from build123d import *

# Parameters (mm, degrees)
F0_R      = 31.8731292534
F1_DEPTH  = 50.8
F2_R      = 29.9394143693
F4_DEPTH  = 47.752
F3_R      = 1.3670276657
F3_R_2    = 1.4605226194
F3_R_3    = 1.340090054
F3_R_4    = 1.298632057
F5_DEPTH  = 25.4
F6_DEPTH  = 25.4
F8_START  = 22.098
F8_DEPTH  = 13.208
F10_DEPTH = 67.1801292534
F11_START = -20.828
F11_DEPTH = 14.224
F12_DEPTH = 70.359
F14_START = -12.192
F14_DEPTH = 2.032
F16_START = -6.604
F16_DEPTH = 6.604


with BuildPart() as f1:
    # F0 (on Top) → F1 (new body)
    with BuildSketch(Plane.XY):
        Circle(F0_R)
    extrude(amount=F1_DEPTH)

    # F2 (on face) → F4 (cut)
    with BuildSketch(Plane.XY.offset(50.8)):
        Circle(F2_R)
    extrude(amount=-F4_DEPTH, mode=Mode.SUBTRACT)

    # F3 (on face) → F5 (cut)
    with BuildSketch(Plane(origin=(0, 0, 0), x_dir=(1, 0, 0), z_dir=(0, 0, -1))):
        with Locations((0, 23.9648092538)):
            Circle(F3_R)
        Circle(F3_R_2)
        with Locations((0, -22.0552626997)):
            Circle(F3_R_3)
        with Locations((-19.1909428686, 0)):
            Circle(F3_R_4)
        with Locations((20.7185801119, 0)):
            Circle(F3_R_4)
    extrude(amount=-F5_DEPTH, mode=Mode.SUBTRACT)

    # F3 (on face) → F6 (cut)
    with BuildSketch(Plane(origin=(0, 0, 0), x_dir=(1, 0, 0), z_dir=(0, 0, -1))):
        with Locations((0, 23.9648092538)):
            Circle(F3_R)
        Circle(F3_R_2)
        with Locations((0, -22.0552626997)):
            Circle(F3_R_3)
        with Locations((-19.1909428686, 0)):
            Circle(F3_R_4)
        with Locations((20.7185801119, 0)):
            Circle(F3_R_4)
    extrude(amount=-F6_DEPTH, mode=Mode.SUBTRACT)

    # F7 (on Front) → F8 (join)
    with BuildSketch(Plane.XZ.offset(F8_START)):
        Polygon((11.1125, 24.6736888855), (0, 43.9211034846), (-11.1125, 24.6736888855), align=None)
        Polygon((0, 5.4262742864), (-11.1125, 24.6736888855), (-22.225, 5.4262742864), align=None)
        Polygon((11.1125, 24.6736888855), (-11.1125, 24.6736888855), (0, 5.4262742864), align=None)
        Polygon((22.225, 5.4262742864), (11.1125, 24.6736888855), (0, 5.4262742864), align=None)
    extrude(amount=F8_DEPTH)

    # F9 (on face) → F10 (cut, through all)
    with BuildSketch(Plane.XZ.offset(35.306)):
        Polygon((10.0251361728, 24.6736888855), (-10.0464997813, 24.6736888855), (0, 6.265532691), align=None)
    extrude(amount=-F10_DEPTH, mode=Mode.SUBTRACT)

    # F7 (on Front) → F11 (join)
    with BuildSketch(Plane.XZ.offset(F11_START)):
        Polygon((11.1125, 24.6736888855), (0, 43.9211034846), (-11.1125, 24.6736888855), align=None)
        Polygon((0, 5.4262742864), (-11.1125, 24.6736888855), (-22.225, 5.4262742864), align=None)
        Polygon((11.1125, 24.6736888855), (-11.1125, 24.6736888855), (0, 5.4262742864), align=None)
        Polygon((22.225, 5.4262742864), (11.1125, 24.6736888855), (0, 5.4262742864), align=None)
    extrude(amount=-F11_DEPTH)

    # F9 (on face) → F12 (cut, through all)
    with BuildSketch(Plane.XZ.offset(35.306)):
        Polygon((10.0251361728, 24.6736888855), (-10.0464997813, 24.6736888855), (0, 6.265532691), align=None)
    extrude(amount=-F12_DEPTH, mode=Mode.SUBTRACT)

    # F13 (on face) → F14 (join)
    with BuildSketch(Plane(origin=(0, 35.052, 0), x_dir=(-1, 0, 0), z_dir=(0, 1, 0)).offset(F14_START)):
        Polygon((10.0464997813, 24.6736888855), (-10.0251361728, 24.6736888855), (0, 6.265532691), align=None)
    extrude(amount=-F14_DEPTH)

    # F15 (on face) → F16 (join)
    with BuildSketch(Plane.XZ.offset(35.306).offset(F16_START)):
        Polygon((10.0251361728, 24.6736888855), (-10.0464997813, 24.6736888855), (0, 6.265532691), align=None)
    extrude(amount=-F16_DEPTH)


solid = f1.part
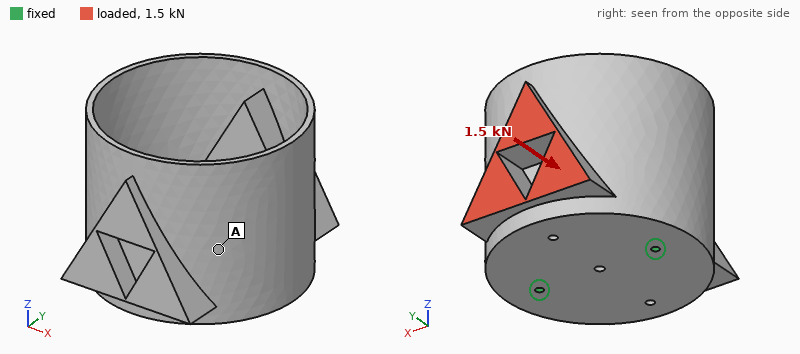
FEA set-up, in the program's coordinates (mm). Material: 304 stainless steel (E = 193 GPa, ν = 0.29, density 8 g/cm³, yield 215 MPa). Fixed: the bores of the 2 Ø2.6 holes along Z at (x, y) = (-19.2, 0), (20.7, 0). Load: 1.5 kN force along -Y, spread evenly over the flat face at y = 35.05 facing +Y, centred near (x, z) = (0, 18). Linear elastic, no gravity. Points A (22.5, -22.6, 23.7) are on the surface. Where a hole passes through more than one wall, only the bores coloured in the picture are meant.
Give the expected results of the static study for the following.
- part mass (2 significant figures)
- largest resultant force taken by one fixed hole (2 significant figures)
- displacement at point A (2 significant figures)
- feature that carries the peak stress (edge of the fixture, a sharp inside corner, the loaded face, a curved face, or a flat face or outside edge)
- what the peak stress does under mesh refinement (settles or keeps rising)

350 g
790 N
0.15 mm
edge of the fixture
keeps rising
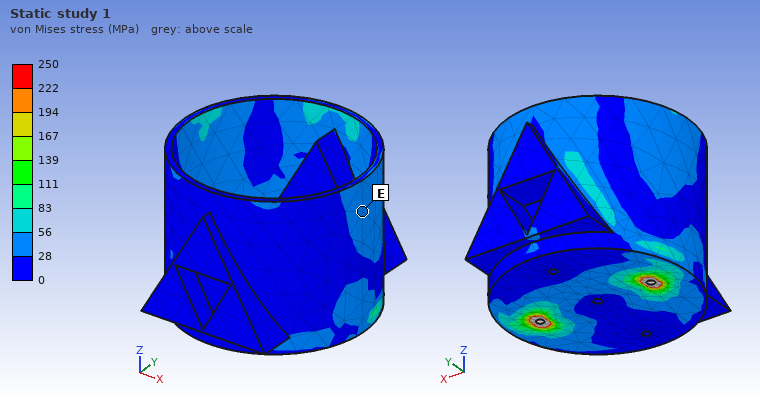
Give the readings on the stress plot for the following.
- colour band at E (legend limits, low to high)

28 to 56 MPa
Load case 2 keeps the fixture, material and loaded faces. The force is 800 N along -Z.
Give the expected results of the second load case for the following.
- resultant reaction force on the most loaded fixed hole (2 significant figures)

420 N
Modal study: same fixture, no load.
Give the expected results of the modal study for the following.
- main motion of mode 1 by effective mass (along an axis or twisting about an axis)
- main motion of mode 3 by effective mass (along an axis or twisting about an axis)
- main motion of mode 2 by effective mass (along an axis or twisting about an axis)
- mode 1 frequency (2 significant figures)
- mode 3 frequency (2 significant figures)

along Y
along X
along Z
570 Hz
2200 Hz
